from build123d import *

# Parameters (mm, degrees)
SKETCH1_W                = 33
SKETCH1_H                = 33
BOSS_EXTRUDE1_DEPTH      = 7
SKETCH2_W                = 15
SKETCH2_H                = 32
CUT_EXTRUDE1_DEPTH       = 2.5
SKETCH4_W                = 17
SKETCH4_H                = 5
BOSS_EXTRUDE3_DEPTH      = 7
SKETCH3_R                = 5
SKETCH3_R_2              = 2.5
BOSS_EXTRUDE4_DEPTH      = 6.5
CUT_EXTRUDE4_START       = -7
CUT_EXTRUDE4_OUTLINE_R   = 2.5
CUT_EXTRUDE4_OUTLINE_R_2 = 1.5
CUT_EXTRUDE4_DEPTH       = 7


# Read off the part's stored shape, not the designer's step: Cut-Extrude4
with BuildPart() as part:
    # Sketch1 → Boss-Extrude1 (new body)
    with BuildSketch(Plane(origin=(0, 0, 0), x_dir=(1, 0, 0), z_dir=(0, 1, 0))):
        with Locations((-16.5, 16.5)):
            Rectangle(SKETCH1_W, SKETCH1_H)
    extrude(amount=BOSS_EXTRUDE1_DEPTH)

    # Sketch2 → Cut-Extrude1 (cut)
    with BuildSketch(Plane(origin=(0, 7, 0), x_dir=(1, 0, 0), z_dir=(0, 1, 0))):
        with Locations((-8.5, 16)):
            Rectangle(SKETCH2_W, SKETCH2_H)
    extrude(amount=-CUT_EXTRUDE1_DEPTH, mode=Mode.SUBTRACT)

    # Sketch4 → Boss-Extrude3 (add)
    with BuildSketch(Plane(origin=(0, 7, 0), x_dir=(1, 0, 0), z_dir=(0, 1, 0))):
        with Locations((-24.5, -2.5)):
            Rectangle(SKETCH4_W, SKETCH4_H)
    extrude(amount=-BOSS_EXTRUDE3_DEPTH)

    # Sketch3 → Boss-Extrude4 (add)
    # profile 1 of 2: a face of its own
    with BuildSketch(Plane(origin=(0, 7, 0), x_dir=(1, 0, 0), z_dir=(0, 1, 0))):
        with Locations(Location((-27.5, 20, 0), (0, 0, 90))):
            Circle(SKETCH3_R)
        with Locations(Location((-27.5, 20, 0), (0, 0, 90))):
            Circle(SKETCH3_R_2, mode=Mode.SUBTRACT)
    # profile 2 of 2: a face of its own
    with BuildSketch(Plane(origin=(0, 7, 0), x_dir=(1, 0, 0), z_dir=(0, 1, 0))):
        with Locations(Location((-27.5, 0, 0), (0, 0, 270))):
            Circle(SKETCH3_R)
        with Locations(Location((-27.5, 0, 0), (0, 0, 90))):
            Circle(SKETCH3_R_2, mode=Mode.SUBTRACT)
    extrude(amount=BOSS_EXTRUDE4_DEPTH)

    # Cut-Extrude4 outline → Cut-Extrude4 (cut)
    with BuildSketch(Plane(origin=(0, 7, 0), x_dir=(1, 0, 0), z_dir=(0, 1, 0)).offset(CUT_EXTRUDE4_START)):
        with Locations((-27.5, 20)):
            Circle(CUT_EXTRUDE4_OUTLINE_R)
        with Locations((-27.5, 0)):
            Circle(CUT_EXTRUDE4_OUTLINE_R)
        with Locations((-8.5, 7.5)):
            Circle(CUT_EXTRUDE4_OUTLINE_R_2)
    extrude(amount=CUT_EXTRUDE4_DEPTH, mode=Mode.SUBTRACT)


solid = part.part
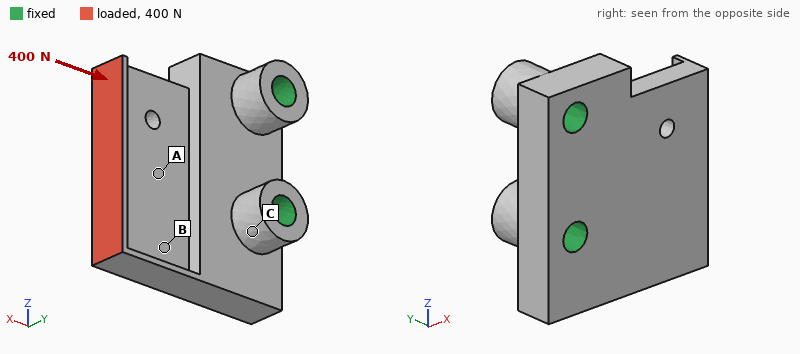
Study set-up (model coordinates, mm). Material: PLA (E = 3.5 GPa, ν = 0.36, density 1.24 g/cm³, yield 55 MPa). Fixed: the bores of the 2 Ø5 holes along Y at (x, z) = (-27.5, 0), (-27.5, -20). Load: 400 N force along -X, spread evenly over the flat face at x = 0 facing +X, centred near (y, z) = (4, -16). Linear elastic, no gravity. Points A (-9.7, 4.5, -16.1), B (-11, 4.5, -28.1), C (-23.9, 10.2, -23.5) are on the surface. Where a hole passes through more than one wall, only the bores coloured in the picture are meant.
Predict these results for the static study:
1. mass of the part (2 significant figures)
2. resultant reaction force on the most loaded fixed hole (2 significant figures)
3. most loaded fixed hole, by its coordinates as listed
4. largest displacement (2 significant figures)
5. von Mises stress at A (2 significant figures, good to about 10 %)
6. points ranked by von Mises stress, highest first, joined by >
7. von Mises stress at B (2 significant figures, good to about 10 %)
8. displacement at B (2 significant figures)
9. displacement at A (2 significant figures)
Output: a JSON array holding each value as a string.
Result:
["9.3 g", "310 N", "(-27.5, -20)", "0.15 mm", "6.9 MPa", "A > B > C", "5.6 MPa", "0.026 mm", "0.027 mm"]
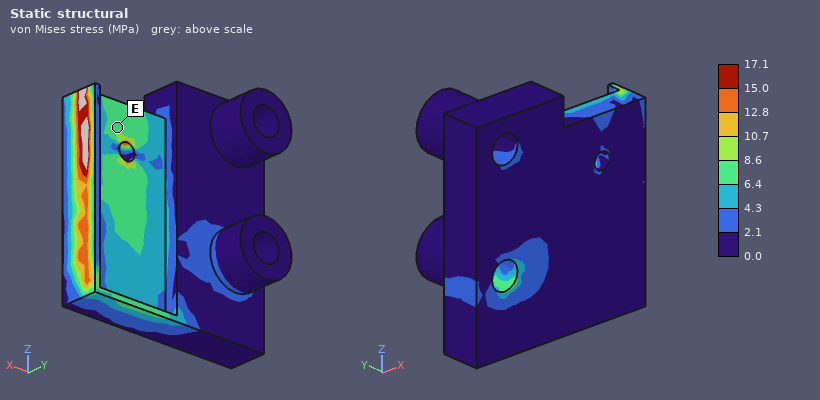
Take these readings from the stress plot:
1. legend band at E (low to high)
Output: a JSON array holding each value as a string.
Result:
["6.4 to 8.6 MPa"]
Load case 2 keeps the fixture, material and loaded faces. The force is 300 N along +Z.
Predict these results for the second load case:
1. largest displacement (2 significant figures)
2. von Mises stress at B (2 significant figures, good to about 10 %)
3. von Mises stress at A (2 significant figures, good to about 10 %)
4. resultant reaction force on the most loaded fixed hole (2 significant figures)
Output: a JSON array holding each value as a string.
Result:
["0.16 mm", "4.0 MPa", "8.1 MPa", "380 N"]
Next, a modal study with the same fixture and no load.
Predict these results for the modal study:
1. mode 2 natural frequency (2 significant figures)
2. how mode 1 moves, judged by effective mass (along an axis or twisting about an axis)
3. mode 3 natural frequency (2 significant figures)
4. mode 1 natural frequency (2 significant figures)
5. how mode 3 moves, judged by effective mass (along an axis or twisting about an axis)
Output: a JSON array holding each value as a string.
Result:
["4100 Hz", "along Y", "6600 Hz", "2600 Hz", "along Z"]
